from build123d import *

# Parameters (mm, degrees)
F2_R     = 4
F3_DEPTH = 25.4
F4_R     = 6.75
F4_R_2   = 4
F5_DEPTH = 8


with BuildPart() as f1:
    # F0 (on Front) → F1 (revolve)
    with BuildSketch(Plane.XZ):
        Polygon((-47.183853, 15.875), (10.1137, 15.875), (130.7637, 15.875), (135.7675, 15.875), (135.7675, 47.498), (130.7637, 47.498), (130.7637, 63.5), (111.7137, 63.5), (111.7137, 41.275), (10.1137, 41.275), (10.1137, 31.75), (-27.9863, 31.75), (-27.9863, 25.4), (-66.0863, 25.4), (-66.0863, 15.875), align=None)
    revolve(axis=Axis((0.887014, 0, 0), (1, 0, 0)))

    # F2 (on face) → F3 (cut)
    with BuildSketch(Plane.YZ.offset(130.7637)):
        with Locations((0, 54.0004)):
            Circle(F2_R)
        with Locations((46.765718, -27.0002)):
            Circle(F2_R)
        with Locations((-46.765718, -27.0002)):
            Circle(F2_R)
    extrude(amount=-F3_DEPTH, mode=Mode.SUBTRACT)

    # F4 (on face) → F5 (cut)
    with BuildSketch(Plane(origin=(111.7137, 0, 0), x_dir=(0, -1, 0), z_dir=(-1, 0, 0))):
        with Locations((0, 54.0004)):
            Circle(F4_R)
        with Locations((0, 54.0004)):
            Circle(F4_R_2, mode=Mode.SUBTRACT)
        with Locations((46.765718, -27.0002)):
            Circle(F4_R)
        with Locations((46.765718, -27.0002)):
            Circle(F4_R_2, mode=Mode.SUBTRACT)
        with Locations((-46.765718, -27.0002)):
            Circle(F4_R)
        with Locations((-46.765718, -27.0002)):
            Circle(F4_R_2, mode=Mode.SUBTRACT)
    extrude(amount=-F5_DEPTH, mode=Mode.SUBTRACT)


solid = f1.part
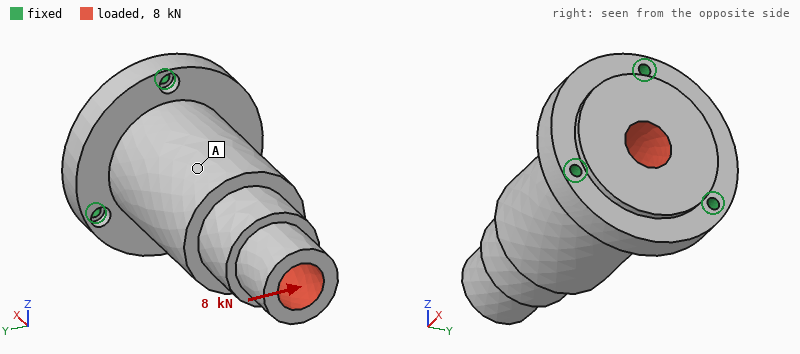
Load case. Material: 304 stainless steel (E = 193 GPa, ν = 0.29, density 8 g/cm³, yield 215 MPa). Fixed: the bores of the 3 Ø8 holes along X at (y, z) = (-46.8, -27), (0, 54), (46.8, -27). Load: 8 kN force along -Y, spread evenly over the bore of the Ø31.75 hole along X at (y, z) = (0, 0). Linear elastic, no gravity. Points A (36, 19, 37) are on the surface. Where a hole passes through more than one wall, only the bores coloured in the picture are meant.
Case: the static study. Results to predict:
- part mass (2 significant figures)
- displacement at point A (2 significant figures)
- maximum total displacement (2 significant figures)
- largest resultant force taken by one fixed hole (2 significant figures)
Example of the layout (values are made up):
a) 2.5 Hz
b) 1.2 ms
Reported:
a) 6.8 kg
b) 18 µm
c) 45 µm
d) 8.6 kN
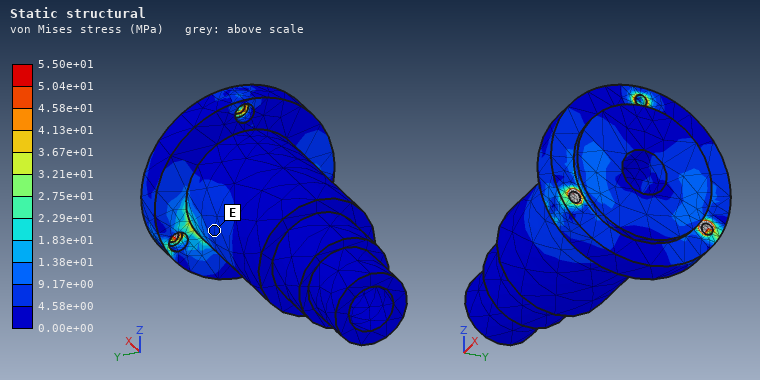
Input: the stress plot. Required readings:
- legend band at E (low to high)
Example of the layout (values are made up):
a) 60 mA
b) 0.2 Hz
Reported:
a) 4.58e+00 to 9.17e+00 MPa
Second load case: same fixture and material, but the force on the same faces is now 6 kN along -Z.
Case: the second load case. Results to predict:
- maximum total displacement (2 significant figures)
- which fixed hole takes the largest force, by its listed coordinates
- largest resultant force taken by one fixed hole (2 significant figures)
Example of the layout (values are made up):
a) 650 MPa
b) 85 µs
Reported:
a) 33 µm
b) (0, 54)
c) 7.5 kN
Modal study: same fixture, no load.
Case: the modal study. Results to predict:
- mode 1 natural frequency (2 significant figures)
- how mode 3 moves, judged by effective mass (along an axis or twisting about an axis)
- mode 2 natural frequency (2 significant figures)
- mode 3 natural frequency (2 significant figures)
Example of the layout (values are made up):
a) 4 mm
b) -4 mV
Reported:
a) 1400 Hz
b) along X
c) 1400 Hz
d) 3700 Hz
